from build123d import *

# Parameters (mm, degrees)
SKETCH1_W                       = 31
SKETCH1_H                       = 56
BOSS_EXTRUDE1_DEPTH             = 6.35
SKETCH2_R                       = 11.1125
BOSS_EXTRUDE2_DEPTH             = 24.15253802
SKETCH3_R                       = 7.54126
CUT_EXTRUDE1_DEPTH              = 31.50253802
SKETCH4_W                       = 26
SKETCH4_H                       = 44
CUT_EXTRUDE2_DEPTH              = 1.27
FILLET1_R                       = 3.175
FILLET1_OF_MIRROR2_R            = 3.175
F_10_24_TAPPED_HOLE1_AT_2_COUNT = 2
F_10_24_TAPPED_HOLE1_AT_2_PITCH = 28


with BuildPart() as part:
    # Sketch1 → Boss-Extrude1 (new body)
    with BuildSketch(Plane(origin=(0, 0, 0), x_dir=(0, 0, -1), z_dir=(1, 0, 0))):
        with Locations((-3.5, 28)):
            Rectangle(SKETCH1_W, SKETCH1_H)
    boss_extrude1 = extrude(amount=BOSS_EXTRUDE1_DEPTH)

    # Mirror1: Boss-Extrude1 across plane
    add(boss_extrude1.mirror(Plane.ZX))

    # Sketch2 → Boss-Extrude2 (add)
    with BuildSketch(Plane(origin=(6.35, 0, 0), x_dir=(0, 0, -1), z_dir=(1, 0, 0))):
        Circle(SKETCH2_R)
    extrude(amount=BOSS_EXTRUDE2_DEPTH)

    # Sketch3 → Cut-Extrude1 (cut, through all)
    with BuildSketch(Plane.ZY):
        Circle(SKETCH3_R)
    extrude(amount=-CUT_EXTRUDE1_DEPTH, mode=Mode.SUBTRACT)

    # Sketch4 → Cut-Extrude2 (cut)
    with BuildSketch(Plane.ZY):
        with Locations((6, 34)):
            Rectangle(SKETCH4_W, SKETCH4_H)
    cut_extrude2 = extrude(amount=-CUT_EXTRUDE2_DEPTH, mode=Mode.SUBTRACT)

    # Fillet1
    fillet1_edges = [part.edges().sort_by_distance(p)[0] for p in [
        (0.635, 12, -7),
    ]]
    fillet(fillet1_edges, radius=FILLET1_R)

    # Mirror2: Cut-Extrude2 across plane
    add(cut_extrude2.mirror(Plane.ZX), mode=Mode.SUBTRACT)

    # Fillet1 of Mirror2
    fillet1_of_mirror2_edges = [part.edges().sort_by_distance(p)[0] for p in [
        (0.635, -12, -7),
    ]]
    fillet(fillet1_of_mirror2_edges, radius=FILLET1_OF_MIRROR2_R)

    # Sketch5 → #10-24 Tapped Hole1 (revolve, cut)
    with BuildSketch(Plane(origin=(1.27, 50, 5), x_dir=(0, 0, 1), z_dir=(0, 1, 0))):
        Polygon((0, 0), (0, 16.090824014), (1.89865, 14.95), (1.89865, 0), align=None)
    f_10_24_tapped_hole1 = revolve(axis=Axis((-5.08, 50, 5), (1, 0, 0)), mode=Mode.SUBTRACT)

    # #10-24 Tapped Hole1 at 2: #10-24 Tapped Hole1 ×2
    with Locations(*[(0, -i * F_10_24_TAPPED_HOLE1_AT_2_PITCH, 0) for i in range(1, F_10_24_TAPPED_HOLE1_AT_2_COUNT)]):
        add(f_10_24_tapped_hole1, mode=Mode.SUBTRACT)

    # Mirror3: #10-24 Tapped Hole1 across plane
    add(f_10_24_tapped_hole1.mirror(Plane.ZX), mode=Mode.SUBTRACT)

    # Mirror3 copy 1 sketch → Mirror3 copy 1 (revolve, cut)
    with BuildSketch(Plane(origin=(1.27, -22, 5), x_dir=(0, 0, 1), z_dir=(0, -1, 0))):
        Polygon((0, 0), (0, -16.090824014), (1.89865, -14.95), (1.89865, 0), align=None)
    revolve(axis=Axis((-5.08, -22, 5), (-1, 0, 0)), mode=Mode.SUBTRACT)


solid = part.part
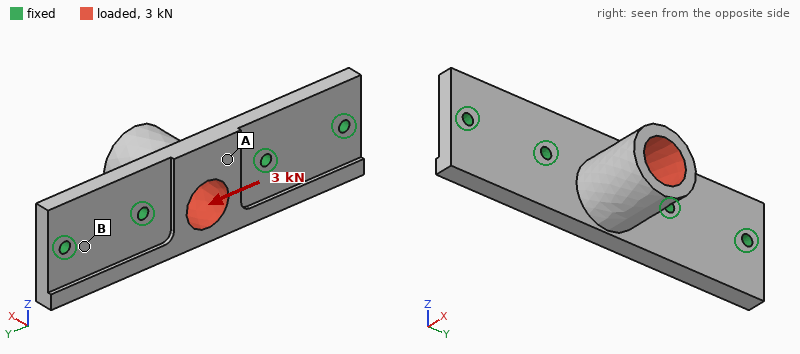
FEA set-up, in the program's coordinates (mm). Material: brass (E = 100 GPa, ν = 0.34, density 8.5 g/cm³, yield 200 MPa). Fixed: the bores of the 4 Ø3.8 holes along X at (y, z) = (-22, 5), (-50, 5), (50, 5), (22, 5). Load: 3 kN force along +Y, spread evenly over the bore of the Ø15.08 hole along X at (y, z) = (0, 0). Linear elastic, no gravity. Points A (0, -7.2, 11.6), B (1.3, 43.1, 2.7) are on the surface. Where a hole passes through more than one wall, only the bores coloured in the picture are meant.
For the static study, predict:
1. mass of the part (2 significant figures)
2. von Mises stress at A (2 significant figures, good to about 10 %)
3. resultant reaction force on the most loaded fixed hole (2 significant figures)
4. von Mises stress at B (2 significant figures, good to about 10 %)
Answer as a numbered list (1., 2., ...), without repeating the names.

1. 190 g
2. 21 MPa
3. 1.6 kN
4. 7.0 MPa
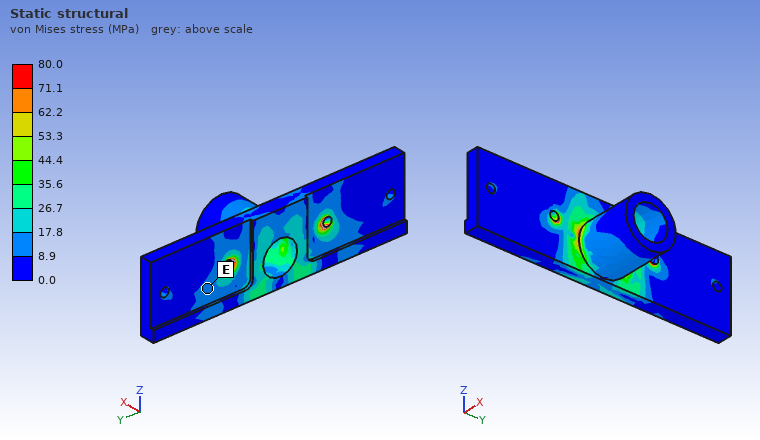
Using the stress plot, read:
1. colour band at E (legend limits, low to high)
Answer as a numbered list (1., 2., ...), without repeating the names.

1. 8.9 to 17.8 MPa
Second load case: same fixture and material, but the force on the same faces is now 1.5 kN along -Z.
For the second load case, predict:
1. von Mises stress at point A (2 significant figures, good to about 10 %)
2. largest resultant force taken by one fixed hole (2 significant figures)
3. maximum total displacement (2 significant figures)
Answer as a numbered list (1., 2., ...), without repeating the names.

1. 20 MPa
2. 850 N
3. 84 µm
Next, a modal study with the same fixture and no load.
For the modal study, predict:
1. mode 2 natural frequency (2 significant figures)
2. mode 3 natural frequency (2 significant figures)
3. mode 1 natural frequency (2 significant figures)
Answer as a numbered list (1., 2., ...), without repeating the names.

1. 6300 Hz
2. 6500 Hz
3. 3100 Hz
